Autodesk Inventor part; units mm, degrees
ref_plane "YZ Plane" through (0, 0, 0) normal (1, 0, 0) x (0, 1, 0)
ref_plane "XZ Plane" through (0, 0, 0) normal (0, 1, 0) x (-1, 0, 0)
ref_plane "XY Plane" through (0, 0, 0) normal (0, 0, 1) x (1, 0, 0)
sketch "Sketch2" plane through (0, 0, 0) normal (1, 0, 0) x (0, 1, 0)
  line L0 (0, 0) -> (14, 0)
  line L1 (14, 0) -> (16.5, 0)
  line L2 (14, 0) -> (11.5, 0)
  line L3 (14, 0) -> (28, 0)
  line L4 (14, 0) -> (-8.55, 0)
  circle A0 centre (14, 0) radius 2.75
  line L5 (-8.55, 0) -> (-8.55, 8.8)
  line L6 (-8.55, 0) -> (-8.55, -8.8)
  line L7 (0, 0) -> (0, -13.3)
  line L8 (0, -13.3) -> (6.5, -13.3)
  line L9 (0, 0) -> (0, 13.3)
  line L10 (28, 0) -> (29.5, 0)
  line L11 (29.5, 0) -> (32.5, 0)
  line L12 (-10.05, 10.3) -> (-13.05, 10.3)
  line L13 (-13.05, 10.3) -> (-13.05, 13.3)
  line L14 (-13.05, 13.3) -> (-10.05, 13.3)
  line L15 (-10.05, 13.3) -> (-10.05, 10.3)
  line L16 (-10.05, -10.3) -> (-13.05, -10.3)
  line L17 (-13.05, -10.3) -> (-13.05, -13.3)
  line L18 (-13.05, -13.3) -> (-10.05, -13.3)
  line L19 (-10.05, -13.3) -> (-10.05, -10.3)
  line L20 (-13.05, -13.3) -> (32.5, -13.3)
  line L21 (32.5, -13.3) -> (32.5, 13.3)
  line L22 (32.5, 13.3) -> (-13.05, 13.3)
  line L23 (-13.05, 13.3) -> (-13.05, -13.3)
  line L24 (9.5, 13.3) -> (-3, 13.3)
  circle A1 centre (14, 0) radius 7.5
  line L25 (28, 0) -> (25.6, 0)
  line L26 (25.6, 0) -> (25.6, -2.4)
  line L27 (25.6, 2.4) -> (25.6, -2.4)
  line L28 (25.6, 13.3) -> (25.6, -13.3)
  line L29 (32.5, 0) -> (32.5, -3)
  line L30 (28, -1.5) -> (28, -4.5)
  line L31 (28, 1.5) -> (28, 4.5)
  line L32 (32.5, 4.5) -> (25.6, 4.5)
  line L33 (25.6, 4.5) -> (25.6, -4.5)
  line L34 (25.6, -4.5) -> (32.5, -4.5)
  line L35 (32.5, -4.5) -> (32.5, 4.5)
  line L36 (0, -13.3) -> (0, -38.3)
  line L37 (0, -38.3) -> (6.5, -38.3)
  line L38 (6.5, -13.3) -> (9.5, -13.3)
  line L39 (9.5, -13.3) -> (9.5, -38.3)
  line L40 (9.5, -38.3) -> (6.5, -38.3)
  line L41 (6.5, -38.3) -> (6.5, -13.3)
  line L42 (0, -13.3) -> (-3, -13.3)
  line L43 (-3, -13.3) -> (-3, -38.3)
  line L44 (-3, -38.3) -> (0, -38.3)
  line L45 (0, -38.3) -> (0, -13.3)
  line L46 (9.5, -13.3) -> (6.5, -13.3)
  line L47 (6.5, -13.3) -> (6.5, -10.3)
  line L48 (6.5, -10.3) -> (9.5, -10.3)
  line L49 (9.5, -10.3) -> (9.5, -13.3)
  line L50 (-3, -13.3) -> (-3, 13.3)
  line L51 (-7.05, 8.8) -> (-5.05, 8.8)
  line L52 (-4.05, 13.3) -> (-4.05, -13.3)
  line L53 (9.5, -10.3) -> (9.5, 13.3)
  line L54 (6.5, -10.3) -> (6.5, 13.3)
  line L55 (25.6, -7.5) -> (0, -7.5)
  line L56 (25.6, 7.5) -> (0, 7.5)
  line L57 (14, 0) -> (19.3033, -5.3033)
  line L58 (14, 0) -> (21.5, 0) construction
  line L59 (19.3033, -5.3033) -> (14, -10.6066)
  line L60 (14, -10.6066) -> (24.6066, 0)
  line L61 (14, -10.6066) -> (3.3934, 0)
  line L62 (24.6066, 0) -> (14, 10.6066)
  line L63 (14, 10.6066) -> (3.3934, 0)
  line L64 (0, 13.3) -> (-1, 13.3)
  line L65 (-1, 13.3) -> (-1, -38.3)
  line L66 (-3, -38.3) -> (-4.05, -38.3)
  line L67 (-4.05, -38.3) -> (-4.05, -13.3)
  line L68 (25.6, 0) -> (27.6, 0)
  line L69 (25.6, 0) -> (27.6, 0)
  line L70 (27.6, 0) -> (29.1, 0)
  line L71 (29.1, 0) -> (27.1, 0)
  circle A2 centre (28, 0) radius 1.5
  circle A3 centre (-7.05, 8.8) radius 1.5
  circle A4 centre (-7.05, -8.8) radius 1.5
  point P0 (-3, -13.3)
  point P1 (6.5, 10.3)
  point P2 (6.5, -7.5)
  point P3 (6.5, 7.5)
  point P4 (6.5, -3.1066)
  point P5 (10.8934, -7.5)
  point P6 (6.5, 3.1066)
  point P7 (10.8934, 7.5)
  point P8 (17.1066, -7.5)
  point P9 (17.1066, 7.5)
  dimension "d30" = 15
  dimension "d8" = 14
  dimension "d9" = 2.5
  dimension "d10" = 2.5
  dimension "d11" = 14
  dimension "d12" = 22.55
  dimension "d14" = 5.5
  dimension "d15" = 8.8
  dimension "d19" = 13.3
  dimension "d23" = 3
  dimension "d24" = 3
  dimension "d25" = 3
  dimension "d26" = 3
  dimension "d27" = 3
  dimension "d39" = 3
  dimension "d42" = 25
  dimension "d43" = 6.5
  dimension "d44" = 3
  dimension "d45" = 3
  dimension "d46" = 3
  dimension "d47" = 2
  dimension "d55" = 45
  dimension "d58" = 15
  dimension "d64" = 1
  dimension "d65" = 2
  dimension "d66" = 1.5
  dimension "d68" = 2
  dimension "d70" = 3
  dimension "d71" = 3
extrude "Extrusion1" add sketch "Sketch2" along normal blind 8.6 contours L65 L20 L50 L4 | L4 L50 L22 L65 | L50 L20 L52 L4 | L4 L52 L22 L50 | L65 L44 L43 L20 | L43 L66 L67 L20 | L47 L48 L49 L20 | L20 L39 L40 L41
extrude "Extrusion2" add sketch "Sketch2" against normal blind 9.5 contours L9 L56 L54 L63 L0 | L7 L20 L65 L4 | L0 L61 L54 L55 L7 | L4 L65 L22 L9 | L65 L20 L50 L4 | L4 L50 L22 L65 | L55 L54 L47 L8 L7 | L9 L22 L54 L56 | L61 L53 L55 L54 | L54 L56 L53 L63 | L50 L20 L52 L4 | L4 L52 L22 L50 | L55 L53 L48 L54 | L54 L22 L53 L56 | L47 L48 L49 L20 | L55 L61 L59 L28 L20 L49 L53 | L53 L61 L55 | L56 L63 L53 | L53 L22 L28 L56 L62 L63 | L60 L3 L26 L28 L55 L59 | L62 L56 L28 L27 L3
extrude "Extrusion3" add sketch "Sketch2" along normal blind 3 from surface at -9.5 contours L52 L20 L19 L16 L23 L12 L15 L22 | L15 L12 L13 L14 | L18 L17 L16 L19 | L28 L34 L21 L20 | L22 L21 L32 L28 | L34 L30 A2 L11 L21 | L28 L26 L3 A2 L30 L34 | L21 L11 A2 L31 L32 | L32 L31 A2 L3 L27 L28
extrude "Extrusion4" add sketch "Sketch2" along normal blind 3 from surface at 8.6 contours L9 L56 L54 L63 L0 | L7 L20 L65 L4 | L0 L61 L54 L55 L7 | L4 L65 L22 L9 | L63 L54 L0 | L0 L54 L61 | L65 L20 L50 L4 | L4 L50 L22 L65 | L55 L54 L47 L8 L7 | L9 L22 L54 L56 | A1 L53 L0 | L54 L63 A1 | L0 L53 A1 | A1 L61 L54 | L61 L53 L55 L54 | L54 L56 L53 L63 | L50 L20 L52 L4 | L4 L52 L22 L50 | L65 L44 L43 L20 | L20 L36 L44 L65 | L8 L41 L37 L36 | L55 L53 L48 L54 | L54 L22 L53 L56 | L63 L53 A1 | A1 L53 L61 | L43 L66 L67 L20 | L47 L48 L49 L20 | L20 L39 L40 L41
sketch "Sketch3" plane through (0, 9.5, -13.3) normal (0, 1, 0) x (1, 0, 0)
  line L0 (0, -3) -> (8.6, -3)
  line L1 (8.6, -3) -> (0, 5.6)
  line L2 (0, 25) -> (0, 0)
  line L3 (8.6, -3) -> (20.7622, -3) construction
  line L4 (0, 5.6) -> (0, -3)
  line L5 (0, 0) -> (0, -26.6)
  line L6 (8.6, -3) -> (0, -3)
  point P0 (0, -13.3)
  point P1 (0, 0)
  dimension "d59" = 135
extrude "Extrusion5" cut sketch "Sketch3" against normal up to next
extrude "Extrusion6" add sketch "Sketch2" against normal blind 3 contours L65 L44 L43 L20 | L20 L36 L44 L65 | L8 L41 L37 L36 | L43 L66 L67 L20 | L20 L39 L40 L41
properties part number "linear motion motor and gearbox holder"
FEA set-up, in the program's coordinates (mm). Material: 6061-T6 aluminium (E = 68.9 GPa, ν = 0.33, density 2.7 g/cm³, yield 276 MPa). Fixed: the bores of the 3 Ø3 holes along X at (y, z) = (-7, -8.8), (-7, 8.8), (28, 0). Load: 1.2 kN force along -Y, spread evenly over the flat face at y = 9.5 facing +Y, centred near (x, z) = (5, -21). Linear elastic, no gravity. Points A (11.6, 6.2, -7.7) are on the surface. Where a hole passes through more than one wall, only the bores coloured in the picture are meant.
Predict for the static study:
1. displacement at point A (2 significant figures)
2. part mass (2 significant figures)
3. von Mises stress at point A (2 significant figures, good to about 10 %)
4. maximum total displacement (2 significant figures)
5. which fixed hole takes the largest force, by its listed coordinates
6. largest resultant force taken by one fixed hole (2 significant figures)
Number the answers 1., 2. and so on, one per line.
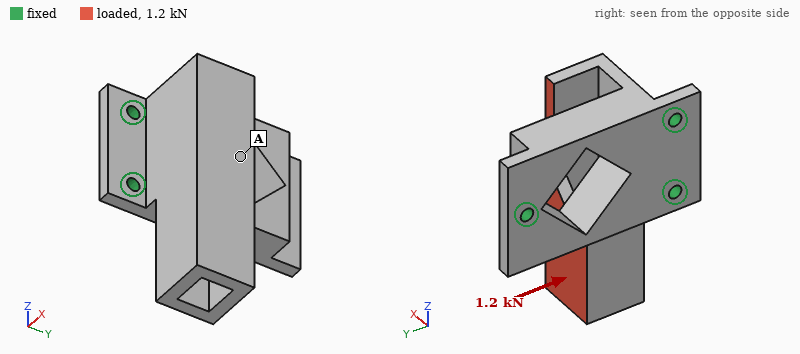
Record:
1. 0.093 mm
2. 31 g
3. 18 MPa
4. 0.16 mm
5. (28, 0)
6. 1.1 kN
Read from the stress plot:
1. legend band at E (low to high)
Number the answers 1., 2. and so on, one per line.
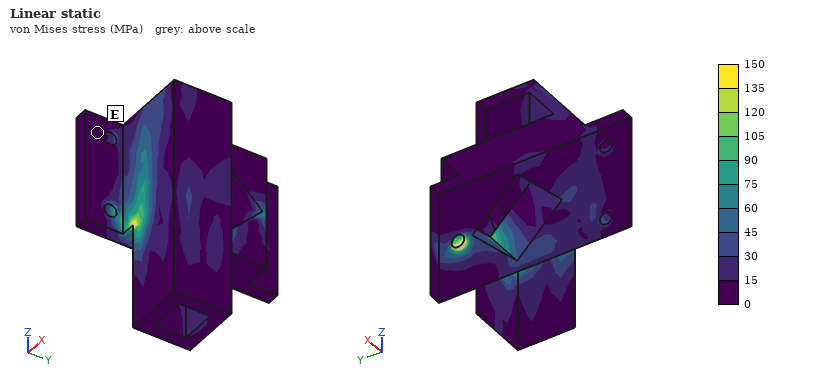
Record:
1. 0 to 15 MPa
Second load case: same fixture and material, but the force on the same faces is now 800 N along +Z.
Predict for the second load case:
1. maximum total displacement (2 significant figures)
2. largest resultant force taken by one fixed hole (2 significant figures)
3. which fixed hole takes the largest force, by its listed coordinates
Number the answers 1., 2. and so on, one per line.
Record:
1. 69 µm
2. 780 N
3. (-7, 8.8)
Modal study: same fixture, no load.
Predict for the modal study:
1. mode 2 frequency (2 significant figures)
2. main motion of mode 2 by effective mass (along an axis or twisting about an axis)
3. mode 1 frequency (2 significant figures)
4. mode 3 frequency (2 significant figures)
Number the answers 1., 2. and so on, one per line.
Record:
1. 5100 Hz
2. along Y
3. 4600 Hz
4. 7300 Hz
